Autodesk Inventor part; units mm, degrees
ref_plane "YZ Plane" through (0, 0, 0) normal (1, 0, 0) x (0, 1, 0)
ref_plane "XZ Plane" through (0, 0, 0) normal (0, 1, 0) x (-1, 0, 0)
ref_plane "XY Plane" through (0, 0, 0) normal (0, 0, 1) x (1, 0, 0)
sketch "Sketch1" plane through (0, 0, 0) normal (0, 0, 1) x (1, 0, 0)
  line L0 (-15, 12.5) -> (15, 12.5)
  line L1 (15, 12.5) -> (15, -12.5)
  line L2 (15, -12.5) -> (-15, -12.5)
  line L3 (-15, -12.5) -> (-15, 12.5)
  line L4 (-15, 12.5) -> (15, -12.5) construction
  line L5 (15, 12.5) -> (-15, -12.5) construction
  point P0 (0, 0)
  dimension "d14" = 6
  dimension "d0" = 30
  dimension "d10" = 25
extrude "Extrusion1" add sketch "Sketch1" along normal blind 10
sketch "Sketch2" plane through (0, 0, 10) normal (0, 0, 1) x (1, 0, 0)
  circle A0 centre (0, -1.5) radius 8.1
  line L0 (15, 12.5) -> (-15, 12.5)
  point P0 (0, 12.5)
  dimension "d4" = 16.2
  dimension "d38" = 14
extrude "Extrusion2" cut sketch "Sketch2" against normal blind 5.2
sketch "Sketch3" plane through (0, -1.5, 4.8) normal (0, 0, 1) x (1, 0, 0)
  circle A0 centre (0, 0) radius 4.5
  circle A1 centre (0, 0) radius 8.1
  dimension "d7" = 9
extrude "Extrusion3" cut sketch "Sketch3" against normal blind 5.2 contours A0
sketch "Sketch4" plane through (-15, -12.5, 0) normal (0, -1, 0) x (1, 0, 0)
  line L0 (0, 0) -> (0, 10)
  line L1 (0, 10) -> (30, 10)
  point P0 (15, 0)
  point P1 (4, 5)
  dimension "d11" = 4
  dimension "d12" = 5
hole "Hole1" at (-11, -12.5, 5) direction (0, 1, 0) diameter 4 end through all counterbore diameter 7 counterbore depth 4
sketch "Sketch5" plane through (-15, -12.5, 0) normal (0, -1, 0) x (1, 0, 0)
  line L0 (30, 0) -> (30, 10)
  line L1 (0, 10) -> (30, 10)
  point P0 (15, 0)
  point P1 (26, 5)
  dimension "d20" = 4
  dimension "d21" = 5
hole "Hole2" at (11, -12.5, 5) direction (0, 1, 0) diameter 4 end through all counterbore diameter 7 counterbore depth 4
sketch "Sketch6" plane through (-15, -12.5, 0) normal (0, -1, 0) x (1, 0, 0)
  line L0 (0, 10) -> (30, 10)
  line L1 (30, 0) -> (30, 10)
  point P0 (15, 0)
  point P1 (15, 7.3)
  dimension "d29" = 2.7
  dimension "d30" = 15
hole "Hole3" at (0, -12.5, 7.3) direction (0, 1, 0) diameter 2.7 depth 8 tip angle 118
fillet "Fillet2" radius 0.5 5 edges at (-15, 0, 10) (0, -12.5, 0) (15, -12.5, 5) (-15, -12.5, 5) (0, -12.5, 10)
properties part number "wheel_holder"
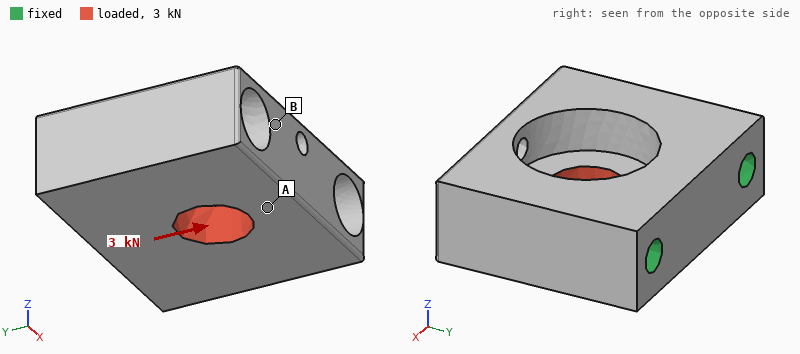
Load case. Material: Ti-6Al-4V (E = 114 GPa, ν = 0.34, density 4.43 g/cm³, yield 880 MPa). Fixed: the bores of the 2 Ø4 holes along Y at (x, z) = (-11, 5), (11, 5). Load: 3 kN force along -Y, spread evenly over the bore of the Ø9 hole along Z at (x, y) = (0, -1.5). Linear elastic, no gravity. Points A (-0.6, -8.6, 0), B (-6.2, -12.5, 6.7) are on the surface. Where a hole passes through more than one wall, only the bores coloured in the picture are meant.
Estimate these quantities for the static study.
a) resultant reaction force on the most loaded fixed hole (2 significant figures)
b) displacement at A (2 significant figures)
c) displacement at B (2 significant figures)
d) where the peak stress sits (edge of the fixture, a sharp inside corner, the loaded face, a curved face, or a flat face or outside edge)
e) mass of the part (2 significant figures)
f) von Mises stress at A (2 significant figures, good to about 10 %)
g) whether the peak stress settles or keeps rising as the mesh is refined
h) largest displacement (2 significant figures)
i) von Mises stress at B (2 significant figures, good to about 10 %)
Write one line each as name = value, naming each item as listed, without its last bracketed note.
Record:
resultant reaction force on the most loaded fixed hole = 1.5 kN
displacement at A = 3.6 µm
displacement at B = 1.4 µm
where the peak stress sits = edge of the fixture
mass of the part = 23 g
von Mises stress at A = 19 MPa
whether the peak stress settles or keeps rising as the mesh is refined = keeps rising
largest displacement = 4.1 µm
von Mises stress at B = 7.3 MPa
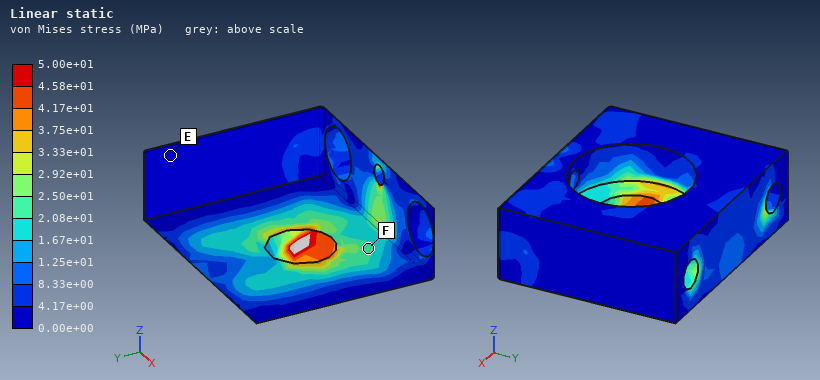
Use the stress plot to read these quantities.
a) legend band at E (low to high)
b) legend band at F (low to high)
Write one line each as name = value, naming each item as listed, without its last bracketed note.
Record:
legend band at E = 0.00e+00 to 4.17e+00 MPa
legend band at F = 2.08e+01 to 2.50e+01 MPa
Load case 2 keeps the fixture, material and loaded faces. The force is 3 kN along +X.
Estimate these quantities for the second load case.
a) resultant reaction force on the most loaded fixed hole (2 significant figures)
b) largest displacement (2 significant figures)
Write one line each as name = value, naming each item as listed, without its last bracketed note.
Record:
resultant reaction force on the most loaded fixed hole = 1.5 kN
largest displacement = 1.9 µm
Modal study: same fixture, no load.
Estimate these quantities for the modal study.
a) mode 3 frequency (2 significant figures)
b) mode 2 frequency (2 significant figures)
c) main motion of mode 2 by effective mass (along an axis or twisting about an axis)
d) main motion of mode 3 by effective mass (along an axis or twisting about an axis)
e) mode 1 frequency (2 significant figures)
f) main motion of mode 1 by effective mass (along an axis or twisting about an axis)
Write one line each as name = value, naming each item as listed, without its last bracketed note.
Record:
mode 3 frequency = 68 kHz
mode 2 frequency = 60 kHz
main motion of mode 2 by effective mass = along Z
main motion of mode 3 by effective mass = along Y
mode 1 frequency = 45 kHz
main motion of mode 1 by effective mass = along Z
